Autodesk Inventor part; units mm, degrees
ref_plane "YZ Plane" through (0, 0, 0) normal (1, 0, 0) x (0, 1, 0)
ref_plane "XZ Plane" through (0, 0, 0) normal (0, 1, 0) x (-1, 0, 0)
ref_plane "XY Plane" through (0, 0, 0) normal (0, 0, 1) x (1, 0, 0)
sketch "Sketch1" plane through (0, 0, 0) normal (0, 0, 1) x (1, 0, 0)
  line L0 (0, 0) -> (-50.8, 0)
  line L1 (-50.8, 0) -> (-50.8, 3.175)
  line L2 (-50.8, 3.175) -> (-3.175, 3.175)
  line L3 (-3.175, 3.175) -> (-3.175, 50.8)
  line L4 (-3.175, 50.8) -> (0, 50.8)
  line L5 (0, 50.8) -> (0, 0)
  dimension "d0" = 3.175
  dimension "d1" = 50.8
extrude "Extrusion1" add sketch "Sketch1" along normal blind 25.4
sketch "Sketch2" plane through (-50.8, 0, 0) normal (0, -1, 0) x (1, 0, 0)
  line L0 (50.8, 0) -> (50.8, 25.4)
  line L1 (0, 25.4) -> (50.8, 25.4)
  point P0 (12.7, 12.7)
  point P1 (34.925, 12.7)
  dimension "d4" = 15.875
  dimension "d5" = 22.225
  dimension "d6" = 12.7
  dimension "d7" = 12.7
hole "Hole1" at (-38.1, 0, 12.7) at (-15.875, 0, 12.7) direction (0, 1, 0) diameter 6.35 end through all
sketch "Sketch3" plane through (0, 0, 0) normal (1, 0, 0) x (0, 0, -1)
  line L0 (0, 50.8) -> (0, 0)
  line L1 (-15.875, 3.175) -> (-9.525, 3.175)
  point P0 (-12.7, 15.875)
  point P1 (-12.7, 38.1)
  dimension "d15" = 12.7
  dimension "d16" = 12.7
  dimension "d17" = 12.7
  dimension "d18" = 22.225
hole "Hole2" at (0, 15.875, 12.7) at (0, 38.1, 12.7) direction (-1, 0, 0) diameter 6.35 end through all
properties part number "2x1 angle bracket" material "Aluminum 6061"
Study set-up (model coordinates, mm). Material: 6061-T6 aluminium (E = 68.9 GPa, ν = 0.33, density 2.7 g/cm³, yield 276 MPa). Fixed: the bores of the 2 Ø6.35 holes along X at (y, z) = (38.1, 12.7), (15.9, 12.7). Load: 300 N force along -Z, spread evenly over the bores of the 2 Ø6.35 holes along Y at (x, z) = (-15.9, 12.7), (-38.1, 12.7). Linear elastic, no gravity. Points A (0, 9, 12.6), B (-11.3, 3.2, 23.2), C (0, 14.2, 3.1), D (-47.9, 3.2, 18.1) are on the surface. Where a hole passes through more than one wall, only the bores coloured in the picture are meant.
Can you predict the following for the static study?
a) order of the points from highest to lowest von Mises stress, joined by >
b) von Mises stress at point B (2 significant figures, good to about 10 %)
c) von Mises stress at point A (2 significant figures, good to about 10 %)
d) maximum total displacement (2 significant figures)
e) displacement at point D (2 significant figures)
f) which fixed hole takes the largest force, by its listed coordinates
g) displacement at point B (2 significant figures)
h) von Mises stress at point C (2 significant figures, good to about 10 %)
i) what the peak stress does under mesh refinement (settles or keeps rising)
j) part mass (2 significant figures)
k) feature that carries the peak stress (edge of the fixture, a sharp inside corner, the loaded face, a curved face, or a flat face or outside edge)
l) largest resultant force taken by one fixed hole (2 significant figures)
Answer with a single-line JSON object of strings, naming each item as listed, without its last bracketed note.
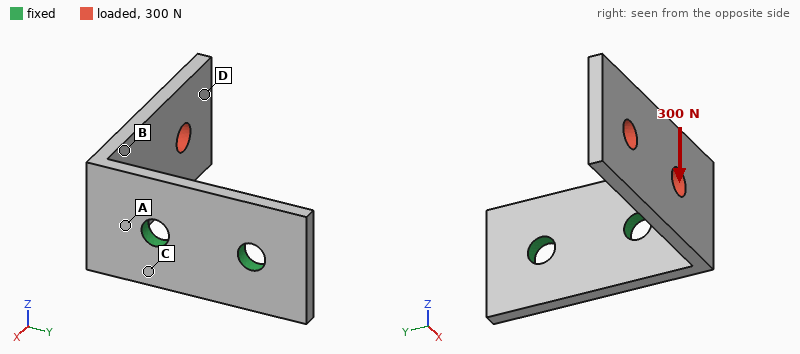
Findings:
{"order of the points from highest to lowest von Mises stress, joined by >": "A > C > B > D", "von Mises stress at point B": "37 MPa", "von Mises stress at point A": "120 MPa", "maximum total displacement": "0.55 mm", "displacement at point D": "0.51 mm", "which fixed hole takes the largest force, by its listed coordinates": "(15.9, 12.7)", "displacement at point B": "0.16 mm", "von Mises stress at point C": "88 MPa", "what the peak stress does under mesh refinement": "keeps rising", "part mass": "20 g", "feature that carries the peak stress": "edge of the fixture", "largest resultant force taken by one fixed hole": "410 N"}
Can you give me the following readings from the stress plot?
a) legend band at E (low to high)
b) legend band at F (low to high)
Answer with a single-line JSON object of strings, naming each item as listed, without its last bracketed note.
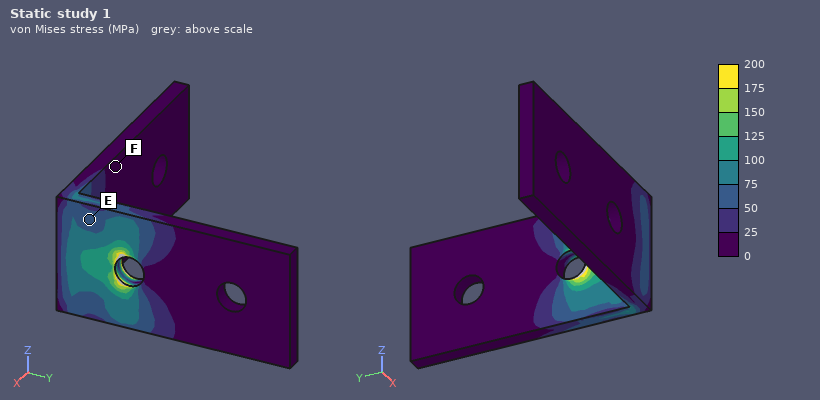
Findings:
{"legend band at E": "50 to 75 MPa", "legend band at F": "0 to 25 MPa"}
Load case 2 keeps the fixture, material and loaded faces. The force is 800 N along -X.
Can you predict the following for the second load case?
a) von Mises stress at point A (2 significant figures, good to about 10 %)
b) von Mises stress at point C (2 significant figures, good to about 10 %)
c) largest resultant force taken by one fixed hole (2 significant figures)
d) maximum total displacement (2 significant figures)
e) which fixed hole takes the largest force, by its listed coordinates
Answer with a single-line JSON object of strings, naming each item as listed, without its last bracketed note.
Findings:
{"von Mises stress at point A": "160 MPa", "von Mises stress at point C": "98 MPa", "largest resultant force taken by one fixed hole": "870 N", "maximum total displacement": "0.71 mm", "which fixed hole takes the largest force, by its listed coordinates": "(15.9, 12.7)"}
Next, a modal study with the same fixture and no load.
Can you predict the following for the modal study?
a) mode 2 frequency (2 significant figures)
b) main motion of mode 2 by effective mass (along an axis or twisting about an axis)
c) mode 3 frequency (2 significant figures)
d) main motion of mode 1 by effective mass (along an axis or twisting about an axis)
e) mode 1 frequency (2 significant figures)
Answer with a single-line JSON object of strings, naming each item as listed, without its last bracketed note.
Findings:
{"mode 2 frequency": "1400 Hz", "main motion of mode 2 by effective mass": "along Z", "mode 3 frequency": "3900 Hz", "main motion of mode 1 by effective mass": "along Y", "mode 1 frequency": "770 Hz"}
